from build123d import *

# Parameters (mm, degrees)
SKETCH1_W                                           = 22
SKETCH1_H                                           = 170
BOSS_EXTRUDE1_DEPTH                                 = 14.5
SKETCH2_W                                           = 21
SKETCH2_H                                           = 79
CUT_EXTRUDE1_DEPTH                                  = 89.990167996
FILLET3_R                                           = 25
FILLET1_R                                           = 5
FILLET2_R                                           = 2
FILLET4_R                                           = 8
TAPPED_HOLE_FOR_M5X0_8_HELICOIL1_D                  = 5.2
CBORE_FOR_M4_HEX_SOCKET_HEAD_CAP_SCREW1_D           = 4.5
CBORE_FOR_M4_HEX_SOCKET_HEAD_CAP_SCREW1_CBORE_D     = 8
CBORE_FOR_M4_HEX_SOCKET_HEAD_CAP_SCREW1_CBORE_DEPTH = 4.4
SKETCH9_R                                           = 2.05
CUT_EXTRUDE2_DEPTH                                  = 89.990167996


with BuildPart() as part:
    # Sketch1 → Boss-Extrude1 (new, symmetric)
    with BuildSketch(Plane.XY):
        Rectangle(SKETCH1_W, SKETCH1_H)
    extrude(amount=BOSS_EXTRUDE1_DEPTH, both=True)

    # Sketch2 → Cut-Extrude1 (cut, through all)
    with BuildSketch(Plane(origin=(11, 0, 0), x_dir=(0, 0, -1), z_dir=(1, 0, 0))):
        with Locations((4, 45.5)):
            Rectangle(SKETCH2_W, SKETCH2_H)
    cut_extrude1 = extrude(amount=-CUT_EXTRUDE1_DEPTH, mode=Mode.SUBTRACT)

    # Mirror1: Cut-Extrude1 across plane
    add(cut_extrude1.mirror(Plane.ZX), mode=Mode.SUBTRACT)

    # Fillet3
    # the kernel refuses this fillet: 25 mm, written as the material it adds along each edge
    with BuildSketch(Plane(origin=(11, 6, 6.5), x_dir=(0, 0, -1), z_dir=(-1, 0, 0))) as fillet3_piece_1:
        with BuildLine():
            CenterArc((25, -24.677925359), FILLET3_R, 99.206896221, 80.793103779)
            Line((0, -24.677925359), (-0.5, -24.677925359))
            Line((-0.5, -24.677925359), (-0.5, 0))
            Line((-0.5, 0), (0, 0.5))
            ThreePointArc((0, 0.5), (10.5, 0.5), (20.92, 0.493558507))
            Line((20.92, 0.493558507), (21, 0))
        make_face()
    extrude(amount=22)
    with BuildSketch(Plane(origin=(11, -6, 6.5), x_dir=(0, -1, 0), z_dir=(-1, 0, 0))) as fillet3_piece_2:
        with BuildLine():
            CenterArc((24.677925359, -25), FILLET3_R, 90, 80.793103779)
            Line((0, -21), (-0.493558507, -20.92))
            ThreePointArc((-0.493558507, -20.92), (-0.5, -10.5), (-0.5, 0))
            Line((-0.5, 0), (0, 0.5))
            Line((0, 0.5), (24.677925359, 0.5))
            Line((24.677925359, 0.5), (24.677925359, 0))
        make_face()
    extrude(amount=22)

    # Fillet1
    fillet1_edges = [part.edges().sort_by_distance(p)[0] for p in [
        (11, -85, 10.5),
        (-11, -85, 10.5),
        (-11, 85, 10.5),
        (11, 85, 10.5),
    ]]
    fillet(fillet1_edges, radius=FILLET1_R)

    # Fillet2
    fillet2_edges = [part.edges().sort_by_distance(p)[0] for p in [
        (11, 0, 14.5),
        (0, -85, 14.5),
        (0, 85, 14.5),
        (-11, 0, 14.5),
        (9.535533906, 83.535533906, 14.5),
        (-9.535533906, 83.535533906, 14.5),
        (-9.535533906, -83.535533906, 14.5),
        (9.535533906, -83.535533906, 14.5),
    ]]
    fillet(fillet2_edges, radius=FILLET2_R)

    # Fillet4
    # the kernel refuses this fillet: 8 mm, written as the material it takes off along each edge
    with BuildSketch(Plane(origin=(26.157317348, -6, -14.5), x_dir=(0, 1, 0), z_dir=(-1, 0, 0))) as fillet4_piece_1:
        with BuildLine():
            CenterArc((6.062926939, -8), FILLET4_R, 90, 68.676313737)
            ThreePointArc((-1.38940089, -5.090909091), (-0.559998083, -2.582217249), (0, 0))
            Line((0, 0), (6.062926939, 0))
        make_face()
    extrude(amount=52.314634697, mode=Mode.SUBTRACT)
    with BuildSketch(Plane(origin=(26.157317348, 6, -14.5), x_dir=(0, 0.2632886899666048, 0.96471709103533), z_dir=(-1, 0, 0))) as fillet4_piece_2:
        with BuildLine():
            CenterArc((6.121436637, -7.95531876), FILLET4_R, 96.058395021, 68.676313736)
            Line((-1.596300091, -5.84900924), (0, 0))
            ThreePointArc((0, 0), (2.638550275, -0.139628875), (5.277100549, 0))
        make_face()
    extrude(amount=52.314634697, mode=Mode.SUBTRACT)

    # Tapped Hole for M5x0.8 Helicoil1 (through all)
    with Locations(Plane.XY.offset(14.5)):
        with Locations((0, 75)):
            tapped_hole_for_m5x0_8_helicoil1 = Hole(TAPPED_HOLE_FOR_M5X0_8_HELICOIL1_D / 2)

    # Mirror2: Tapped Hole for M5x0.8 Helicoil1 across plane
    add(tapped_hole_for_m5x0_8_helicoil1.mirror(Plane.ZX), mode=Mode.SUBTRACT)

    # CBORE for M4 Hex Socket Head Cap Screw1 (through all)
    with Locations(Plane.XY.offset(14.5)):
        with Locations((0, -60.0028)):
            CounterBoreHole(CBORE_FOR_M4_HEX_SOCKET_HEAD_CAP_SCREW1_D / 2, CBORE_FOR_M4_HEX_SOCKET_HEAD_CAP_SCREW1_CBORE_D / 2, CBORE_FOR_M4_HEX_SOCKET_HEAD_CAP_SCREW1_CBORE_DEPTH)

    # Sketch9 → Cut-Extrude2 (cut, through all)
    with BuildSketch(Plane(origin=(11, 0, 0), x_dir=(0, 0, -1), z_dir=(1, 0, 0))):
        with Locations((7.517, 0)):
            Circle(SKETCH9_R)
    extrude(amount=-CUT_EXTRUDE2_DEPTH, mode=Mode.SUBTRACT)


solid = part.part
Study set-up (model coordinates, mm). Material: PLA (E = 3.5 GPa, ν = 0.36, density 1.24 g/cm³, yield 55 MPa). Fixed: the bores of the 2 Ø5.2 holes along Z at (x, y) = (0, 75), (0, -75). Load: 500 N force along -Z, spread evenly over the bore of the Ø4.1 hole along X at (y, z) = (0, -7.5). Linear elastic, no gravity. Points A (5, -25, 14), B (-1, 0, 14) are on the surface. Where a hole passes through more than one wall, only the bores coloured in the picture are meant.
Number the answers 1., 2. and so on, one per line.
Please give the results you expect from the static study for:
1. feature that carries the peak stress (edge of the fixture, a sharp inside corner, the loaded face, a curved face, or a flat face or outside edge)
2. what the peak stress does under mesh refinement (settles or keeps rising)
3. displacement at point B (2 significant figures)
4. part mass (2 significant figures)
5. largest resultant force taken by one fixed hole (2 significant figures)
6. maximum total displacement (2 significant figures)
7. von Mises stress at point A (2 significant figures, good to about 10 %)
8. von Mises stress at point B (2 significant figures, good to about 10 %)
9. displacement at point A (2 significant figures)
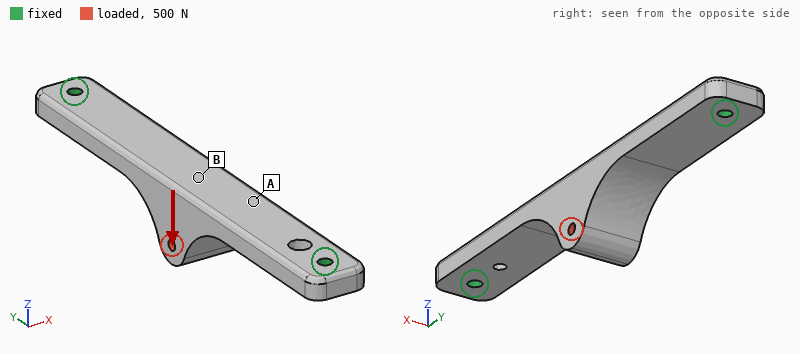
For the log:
1. edge of the fixture
2. keeps rising
3. 1.3 mm
4. 49 g
5. 340 N
6. 1.4 mm
7. 18 MPa
8. 6.6 MPa
9. 1.2 mm
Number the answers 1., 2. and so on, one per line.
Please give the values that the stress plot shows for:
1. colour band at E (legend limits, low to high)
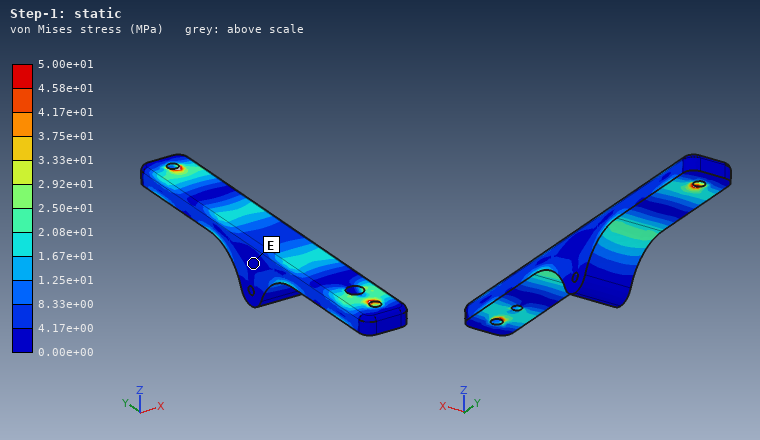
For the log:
1. 0.00e+00 to 4.17e+00 MPa
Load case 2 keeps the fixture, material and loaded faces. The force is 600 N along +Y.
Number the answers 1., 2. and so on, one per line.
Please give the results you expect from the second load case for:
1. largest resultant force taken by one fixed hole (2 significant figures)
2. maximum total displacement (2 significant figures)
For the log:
1. 330 N
2. 0.31 mm
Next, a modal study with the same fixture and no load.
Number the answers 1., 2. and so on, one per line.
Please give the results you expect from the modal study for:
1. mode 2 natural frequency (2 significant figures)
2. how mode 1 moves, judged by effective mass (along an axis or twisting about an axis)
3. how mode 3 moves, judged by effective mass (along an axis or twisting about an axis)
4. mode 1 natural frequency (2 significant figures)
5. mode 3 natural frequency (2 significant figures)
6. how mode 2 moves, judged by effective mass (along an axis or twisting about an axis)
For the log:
1. 760 Hz
2. along Z
3. along X
4. 570 Hz
5. 1300 Hz
6. along X
